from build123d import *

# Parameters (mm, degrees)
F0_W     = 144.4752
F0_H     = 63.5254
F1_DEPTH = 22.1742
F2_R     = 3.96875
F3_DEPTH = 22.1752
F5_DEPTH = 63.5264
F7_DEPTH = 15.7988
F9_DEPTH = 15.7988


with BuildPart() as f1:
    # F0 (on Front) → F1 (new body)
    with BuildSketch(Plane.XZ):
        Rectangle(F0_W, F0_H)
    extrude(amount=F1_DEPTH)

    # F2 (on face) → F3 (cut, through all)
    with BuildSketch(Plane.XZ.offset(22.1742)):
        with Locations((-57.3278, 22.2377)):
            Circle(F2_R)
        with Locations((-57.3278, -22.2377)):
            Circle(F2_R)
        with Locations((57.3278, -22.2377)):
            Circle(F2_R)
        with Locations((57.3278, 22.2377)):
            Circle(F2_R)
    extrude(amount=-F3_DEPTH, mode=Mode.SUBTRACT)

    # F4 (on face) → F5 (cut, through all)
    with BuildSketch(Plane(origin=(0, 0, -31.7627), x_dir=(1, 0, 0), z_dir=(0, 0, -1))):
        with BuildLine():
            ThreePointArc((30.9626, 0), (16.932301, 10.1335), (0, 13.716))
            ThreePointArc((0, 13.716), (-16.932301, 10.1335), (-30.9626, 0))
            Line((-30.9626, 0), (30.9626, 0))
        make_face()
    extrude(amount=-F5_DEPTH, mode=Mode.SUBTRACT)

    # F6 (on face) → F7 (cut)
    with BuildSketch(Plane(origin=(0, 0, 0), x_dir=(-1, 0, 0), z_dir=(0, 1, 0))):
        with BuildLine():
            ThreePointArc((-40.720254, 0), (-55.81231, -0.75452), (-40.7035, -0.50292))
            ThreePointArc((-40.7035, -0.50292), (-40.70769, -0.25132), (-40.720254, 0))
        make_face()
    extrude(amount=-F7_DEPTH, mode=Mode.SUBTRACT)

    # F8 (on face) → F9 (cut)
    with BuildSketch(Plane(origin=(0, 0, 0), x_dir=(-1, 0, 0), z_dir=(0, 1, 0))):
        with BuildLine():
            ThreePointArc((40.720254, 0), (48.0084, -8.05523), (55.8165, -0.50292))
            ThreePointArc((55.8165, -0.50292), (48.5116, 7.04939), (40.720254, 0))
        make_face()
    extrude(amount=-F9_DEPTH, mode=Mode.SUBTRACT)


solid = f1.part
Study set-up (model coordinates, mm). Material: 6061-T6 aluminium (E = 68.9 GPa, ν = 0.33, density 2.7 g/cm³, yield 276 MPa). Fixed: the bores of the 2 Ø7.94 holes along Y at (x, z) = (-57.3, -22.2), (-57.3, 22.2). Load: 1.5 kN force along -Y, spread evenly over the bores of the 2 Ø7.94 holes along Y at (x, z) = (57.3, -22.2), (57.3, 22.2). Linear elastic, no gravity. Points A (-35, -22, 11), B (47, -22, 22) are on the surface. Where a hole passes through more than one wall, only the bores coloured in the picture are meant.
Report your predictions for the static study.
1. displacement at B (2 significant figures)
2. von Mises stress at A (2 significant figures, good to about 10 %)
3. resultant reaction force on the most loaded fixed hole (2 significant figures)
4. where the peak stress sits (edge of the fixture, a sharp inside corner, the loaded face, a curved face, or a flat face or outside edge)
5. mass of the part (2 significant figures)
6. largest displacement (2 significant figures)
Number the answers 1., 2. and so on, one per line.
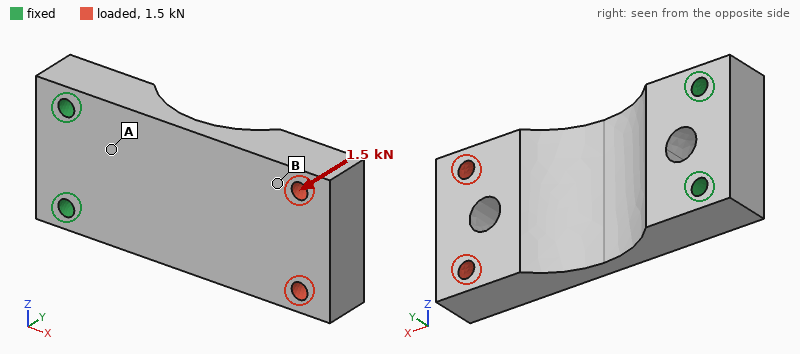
1. 0.69 mm
2. 32 MPa
3. 760 N
4. a flat face or outside edge
5. 420 g
6. 1.0 mm
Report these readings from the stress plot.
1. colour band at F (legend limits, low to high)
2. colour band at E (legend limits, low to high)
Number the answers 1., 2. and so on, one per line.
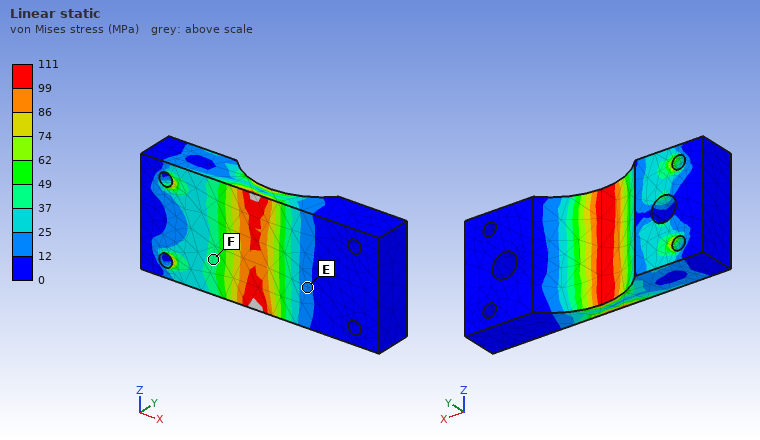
1. 37 to 49 MPa
2. 12 to 25 MPa
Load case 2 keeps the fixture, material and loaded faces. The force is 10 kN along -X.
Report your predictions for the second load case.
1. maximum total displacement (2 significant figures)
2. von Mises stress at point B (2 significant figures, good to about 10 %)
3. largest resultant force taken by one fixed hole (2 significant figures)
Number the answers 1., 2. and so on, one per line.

1. 0.60 mm
2. 8.8 MPa
3. 5.1 kN
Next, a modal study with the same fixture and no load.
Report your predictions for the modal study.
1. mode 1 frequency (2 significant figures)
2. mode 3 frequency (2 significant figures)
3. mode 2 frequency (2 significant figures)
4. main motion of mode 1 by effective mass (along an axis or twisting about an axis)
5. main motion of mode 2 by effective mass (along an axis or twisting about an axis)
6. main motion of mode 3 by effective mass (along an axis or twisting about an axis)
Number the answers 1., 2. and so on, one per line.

1. 580 Hz
2. 2700 Hz
3. 2000 Hz
4. along Y
5. along Z
6. along Z
